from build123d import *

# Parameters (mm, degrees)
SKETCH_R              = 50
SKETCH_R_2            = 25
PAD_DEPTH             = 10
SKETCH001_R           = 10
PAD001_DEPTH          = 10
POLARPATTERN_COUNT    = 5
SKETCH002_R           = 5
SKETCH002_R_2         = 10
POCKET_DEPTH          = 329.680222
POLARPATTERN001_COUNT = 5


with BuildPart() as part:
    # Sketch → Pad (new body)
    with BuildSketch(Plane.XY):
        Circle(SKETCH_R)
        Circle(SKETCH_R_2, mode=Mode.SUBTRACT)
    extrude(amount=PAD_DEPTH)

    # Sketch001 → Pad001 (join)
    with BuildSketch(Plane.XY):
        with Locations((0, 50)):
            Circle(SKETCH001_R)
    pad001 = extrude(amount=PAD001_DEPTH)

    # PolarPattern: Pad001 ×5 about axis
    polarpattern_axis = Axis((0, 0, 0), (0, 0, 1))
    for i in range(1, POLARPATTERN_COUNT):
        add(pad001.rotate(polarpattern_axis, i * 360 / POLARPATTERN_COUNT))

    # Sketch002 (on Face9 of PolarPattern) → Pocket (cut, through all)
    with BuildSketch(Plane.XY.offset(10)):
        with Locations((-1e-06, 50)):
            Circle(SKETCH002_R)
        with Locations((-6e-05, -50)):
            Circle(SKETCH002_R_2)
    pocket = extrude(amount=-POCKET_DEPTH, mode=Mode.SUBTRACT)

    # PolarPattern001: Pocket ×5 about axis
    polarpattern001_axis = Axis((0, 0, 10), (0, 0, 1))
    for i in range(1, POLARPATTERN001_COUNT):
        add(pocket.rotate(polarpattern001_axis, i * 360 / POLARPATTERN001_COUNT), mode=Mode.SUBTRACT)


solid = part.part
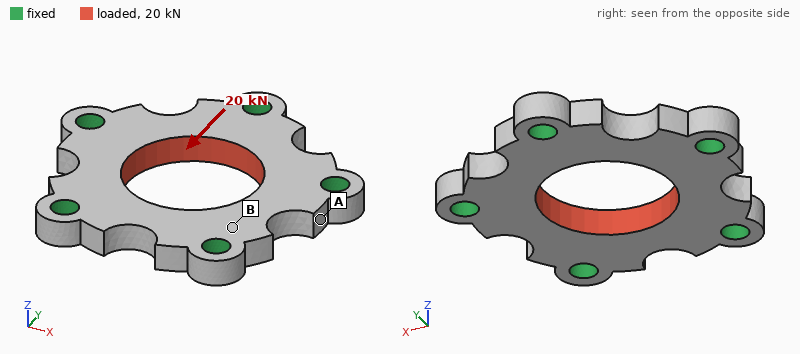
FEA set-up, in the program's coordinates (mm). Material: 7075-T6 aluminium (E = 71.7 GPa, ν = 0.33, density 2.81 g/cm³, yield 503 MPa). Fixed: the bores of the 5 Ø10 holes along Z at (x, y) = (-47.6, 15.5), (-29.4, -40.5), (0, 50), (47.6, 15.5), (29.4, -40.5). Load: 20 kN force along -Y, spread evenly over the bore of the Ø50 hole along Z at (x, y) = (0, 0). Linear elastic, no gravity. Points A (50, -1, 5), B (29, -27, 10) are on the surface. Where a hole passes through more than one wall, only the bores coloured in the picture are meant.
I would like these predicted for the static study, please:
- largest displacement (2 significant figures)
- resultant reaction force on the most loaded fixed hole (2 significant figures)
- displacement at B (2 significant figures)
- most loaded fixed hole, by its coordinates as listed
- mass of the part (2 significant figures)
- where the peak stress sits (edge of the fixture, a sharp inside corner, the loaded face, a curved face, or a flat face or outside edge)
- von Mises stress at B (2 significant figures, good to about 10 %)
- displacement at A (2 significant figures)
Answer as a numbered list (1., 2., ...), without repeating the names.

1. 12 µm
2. 6.1 kN
3. 2.6 µm
4. (0, 50)
5. 160 g
6. edge of the fixture
7. 20 MPa
8. 2.0 µm
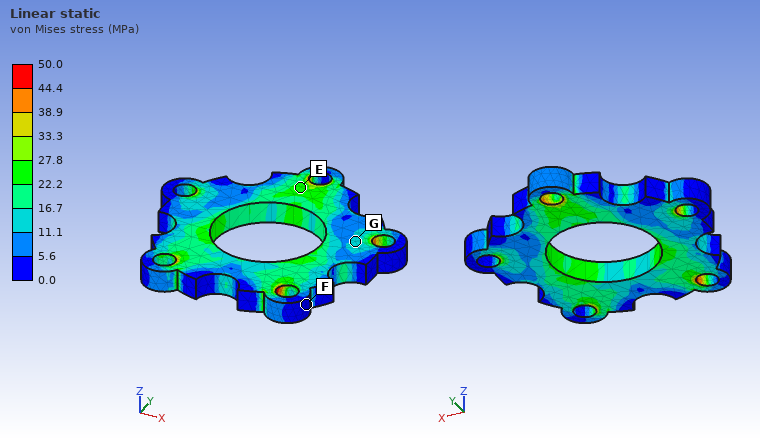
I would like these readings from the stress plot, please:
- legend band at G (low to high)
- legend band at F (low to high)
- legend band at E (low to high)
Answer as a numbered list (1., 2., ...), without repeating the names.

1. 11.1 to 16.7 MPa
2. 0.0 to 5.6 MPa
3. 22.2 to 27.8 MPa
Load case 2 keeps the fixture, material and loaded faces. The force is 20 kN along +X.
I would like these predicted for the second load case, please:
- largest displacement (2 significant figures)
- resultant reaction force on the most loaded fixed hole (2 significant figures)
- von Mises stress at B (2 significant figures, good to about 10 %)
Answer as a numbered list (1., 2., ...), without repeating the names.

1. 12 µm
2. 5.8 kN
3. 15 MPa
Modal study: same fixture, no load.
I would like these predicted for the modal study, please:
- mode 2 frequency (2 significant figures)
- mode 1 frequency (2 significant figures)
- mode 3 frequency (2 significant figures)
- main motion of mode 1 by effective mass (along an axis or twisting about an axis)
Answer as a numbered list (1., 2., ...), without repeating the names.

1. 14 kHz
2. 12 kHz
3. 14 kHz
4. along Z
